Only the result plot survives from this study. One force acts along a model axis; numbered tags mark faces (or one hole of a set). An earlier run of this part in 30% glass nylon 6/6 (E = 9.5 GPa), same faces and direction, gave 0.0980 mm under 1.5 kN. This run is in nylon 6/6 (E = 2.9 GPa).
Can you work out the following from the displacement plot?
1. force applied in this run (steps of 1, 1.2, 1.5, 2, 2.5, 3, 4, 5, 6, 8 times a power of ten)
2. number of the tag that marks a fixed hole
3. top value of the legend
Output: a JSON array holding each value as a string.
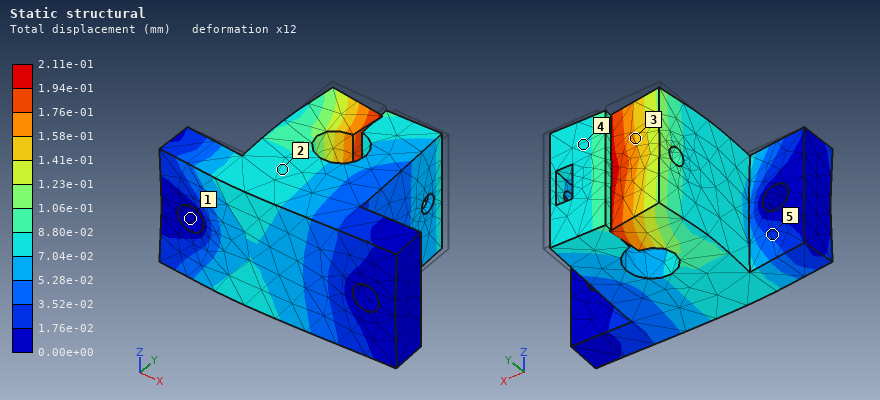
["1 kN", "1", "2.11e-01 mm"]
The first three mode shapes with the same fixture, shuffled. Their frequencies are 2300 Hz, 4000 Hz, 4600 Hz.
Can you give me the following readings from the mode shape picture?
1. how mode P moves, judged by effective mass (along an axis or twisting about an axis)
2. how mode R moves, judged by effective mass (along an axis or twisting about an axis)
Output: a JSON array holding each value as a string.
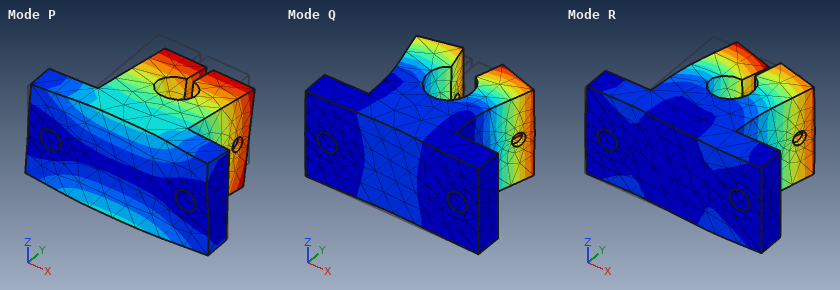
["along Z", "along X"]
